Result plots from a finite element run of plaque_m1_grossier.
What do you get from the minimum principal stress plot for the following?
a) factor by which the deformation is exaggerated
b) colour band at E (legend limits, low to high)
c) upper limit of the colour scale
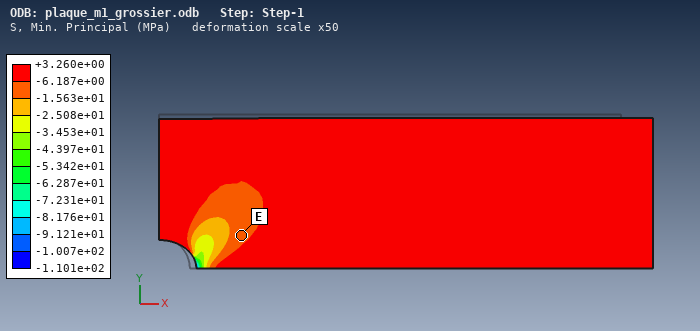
50
-1.563e+01 to -6.187e+00 MPa
+3.260e+00 MPa
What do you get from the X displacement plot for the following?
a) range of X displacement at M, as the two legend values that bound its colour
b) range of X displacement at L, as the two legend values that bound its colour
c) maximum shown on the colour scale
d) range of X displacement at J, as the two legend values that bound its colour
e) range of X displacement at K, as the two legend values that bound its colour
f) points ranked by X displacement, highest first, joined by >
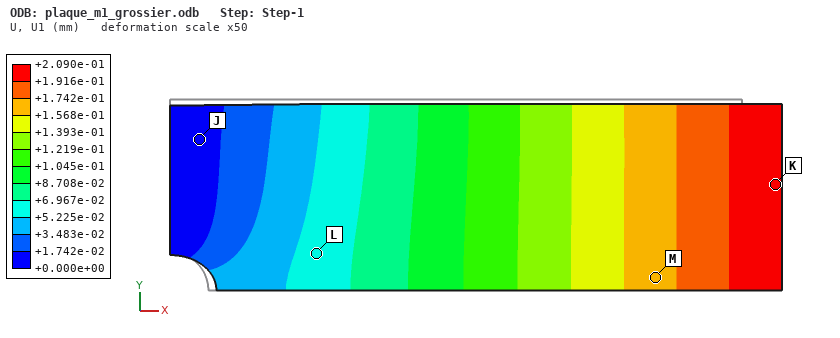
+1.568e-01 to +1.742e-01 mm
+5.225e-02 to +6.967e-02 mm
+2.090e-01 mm
+0.000e+00 to +1.742e-02 mm
+1.916e-01 to +2.090e-01 mm
K > M > L > J
